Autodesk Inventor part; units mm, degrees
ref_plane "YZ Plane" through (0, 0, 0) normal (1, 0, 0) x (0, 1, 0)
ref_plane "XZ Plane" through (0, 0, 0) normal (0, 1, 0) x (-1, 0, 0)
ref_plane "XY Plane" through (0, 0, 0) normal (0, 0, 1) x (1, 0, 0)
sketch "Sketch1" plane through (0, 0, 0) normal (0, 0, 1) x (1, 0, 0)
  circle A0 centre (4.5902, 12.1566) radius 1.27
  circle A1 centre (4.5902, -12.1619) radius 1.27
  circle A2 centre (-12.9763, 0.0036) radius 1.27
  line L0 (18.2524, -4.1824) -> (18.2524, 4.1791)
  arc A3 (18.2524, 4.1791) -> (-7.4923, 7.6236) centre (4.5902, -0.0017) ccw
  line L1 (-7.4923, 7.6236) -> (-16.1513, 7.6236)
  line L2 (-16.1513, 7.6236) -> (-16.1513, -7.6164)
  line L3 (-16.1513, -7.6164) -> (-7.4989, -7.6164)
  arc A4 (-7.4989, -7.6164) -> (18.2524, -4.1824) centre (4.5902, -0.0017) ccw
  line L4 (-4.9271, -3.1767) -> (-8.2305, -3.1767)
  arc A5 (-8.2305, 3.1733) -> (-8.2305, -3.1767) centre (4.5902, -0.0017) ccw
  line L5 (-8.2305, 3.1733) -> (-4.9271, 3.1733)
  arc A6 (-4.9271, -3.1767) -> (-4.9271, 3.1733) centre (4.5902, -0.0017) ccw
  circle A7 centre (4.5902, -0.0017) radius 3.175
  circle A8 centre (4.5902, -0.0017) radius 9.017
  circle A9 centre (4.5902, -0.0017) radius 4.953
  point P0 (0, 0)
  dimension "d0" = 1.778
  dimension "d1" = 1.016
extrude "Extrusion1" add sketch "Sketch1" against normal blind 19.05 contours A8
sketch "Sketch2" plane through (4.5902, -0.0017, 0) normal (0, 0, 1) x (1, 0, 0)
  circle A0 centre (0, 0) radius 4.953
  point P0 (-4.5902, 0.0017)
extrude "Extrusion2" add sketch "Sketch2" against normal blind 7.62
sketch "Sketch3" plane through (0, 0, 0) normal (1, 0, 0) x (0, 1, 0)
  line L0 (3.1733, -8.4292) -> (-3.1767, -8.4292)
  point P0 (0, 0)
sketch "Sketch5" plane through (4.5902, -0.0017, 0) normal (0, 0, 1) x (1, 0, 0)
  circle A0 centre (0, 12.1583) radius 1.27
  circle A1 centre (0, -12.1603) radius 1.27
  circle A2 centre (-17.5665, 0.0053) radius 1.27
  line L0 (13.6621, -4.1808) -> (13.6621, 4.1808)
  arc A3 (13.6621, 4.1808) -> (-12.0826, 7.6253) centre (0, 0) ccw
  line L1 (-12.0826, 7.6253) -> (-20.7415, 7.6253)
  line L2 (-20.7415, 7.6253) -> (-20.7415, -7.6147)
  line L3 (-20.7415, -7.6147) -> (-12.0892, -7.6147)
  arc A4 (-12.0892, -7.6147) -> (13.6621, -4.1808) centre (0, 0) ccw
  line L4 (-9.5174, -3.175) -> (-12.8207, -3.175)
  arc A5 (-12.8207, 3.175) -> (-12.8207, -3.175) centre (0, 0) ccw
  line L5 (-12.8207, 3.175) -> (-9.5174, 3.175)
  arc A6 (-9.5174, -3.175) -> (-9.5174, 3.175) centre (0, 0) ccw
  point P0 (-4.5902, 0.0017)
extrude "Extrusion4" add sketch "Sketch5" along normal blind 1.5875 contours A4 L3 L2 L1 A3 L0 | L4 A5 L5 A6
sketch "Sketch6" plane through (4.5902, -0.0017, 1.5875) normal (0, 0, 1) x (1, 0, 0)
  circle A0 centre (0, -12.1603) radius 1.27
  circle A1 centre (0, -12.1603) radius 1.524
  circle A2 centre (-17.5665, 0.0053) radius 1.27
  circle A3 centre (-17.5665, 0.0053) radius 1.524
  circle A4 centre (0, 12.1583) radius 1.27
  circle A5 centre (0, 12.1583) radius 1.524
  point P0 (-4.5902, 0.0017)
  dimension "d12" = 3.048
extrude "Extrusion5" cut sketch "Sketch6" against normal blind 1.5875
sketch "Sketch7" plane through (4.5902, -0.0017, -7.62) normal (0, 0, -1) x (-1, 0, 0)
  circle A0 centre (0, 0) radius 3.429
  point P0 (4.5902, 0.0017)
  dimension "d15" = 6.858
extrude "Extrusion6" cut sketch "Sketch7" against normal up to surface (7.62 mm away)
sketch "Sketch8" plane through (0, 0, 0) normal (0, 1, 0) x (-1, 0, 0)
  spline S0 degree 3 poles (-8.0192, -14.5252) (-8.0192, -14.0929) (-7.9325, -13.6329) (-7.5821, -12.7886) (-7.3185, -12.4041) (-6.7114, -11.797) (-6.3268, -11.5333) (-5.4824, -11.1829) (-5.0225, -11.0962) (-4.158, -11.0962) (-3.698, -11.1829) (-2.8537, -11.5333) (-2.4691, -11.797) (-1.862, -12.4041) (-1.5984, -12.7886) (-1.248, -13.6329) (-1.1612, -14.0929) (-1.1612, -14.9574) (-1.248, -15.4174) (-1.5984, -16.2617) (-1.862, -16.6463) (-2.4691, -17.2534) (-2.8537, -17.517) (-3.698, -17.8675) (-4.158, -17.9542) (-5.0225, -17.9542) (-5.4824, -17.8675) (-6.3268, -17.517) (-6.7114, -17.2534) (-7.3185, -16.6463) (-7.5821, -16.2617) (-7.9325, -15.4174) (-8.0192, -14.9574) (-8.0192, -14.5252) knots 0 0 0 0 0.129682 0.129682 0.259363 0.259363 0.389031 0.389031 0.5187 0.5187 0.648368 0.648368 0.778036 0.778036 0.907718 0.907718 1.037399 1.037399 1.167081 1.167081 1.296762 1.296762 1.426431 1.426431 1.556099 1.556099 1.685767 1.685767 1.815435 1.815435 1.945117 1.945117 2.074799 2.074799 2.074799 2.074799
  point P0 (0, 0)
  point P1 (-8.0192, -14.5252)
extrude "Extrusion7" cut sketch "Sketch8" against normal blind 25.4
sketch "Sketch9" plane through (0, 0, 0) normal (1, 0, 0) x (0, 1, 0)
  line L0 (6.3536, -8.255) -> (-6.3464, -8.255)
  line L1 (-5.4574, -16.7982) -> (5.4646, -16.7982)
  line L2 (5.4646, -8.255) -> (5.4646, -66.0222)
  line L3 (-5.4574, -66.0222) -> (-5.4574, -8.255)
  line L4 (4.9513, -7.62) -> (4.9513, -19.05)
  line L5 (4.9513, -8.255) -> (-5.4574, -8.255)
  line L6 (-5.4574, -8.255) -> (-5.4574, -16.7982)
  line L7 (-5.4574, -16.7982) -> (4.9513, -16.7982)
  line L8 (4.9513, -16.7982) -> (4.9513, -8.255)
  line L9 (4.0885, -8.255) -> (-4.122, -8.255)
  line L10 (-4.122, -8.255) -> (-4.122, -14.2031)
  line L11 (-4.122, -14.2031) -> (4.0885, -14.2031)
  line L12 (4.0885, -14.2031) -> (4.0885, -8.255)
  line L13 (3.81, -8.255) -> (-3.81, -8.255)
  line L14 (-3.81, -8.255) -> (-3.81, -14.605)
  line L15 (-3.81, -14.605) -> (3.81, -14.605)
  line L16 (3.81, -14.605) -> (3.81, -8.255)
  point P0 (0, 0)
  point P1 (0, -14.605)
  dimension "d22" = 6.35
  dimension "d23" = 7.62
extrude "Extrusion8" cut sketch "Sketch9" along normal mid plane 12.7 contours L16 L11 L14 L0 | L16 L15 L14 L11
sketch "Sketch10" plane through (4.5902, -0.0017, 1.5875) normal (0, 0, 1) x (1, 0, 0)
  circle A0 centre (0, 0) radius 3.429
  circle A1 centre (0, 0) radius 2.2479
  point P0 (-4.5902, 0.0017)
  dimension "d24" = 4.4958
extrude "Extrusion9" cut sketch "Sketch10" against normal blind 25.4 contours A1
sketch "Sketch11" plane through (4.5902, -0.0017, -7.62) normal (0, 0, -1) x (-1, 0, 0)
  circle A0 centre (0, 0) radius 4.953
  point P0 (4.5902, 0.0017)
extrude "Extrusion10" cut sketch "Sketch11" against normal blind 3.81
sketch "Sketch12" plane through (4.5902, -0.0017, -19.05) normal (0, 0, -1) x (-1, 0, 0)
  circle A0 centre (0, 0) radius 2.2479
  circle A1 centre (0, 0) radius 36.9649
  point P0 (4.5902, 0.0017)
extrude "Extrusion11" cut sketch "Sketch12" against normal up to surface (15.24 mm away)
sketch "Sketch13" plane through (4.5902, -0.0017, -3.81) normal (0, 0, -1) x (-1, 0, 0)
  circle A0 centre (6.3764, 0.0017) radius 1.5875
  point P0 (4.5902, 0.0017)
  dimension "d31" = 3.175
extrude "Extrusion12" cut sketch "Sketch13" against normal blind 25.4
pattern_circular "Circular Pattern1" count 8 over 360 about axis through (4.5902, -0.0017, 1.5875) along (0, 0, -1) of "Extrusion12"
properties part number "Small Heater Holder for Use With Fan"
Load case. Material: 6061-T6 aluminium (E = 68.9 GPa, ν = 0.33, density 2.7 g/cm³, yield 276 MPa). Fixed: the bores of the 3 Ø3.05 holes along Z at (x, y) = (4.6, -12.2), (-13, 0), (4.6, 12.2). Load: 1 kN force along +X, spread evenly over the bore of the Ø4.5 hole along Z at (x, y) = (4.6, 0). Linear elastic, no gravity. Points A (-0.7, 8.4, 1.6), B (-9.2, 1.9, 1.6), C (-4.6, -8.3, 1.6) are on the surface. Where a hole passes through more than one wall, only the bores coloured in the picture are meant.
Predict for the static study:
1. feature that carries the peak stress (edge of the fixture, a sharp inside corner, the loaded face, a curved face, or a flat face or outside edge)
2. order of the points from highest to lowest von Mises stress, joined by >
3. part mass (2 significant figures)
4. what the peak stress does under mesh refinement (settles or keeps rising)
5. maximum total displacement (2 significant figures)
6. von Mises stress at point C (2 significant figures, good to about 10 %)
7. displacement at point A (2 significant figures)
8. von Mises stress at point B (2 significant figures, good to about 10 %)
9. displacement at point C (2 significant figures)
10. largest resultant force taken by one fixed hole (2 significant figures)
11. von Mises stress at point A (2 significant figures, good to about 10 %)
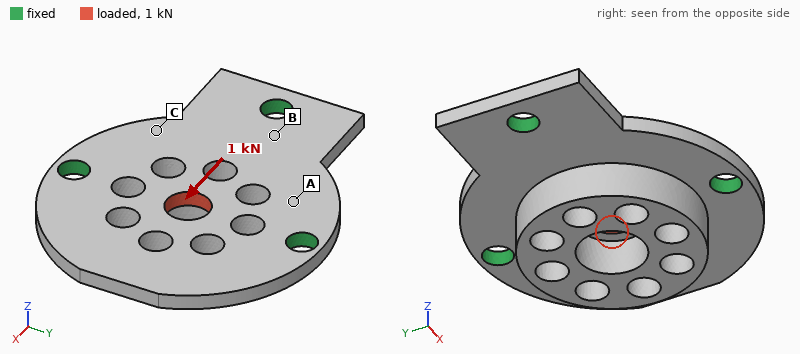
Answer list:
edge of the fixture
B > A > C
4.4 g
keeps rising
9.3 µm
7.1 MPa
2.6 µm
24 MPa
2.6 µm
350 N
16 MPa
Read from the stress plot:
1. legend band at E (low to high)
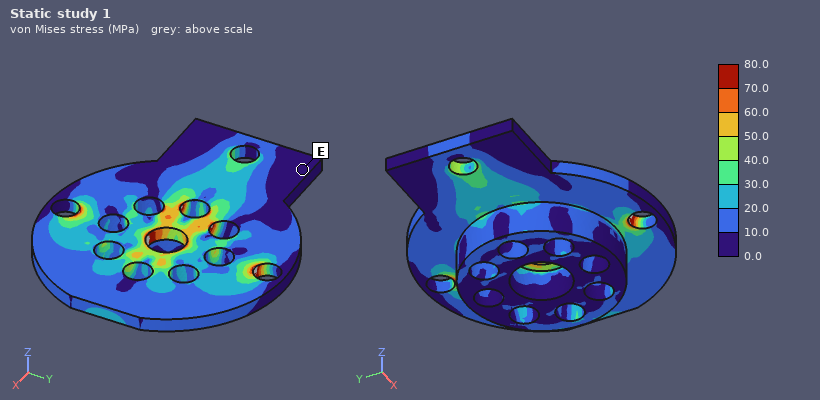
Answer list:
0.0 to 10.0 MPa
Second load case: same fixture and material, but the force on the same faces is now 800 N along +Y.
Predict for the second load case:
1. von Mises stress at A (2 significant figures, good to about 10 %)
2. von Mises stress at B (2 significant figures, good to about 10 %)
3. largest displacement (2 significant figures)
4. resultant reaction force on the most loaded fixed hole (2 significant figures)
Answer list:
8.6 MPa
8.9 MPa
6.3 µm
360 N
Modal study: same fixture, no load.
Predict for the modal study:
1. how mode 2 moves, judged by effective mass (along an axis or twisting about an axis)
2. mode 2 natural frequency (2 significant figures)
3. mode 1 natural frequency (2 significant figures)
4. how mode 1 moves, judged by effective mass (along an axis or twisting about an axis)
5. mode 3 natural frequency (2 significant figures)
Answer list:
along Z
19 kHz
10 kHz
along Z
26 kHz
